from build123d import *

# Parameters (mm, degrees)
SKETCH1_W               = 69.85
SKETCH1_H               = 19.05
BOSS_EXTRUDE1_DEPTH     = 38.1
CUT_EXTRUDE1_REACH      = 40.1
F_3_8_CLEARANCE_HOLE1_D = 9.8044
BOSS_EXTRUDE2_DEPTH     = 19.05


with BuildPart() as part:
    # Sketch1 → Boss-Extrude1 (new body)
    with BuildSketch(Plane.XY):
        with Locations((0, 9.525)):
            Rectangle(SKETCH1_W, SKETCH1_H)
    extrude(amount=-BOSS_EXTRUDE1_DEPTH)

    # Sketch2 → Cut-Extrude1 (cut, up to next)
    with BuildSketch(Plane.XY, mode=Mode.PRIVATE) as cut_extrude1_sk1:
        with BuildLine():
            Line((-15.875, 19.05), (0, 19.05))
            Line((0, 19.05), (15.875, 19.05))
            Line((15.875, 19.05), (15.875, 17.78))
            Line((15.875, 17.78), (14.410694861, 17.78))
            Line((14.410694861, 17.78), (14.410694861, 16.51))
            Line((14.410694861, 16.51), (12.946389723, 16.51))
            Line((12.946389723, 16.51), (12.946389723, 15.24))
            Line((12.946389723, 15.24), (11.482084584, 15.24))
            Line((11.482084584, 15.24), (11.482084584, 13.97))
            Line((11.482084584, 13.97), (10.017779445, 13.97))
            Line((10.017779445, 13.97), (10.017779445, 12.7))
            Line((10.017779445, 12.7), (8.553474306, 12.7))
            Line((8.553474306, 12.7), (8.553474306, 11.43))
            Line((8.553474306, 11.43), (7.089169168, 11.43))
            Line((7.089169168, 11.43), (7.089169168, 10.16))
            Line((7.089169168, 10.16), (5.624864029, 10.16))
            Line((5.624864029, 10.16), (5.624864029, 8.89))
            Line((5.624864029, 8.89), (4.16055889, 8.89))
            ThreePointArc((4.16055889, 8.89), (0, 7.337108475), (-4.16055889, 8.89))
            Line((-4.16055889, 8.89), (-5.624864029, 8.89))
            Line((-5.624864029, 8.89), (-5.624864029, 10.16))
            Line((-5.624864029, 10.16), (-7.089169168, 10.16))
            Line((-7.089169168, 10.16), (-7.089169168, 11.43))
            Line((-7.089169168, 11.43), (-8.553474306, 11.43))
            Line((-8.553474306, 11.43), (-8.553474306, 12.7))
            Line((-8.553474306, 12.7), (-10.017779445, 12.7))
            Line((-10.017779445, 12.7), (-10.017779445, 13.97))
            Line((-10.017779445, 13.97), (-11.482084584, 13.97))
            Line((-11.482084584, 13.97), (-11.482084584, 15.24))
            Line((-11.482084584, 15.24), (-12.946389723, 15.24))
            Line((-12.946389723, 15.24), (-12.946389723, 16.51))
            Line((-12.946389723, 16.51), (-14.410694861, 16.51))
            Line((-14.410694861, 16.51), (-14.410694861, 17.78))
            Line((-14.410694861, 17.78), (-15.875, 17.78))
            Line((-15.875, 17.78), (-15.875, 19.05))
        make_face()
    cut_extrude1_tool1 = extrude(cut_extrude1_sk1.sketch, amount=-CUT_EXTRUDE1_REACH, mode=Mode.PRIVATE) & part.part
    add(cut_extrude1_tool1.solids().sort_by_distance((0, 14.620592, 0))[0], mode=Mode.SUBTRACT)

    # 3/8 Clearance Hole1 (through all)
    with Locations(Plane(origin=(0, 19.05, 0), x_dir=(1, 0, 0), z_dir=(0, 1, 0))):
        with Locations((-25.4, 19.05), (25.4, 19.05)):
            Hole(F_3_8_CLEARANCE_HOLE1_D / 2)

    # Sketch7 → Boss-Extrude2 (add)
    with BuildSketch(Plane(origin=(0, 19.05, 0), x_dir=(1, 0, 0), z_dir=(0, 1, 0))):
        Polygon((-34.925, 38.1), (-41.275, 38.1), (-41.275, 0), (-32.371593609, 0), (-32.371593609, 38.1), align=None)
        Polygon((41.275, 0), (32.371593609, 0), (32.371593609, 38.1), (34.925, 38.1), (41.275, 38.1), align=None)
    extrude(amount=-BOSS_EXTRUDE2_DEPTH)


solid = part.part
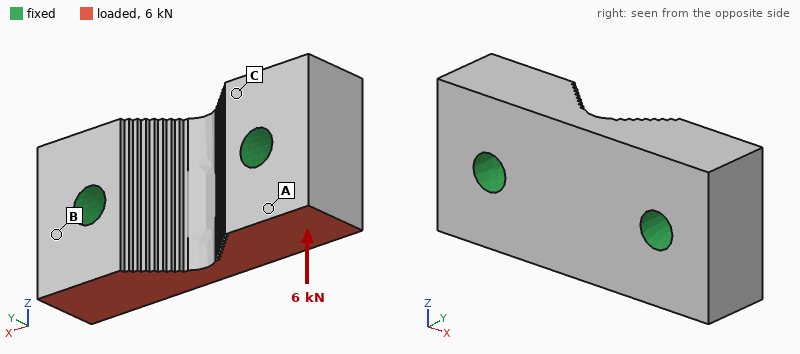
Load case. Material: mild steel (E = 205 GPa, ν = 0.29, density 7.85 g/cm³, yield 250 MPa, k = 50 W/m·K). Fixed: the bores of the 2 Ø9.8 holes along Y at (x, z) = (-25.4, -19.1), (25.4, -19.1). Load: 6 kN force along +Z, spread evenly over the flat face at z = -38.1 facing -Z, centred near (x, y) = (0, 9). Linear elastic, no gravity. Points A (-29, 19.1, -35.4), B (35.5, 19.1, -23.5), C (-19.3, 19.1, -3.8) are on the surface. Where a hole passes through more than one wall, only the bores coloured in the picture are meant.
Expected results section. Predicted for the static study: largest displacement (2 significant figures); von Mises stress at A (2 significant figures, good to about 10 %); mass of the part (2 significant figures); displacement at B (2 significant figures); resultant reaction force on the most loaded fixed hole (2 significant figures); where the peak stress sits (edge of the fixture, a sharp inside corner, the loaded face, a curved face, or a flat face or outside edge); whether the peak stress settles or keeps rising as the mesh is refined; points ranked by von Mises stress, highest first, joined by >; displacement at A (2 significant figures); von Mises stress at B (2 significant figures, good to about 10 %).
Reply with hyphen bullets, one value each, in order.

- 0.92 µm
- 5.4 MPa
- 380 g
- 0.22 µm
- 3.0 kN
- edge of the fixture
- keeps rising
- A > B > C
- 0.34 µm
- 3.0 MPa
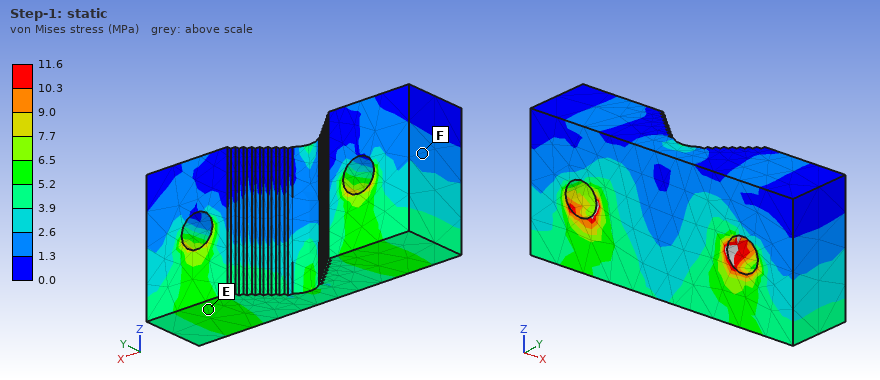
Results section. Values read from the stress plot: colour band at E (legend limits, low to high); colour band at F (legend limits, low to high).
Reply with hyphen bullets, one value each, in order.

- 5.2 to 6.5 MPa
- 1.3 to 2.6 MPa
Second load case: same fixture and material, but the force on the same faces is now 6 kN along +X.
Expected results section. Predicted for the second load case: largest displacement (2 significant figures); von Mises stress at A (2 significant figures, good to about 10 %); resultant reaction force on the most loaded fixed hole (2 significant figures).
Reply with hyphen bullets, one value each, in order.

- 2.7 µm
- 8.7 MPa
- 3.3 kN
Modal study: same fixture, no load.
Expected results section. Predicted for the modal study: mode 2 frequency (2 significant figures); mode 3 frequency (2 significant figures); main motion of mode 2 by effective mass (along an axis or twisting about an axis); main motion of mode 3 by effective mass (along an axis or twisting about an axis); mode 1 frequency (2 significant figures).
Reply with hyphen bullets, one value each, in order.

- 25 kHz
- 26 kHz
- along Y
- twisting about X
- 22 kHz
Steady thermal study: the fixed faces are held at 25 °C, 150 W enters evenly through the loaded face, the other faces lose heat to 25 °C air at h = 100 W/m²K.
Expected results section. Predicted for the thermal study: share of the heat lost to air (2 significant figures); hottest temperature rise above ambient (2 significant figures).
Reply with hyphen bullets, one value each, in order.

- 7.8 %
- 45 K
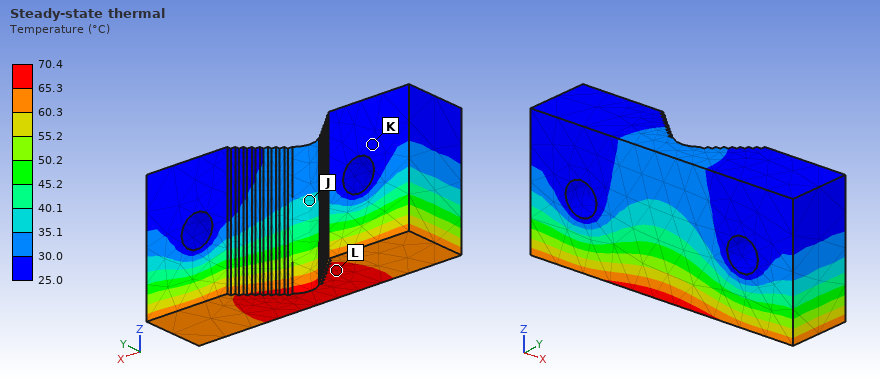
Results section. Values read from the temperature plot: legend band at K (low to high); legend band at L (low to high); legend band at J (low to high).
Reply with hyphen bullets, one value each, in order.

- 25.0 to 30.0 °C
- 65.3 to 70.4 °C
- 35.1 to 40.1 °C
